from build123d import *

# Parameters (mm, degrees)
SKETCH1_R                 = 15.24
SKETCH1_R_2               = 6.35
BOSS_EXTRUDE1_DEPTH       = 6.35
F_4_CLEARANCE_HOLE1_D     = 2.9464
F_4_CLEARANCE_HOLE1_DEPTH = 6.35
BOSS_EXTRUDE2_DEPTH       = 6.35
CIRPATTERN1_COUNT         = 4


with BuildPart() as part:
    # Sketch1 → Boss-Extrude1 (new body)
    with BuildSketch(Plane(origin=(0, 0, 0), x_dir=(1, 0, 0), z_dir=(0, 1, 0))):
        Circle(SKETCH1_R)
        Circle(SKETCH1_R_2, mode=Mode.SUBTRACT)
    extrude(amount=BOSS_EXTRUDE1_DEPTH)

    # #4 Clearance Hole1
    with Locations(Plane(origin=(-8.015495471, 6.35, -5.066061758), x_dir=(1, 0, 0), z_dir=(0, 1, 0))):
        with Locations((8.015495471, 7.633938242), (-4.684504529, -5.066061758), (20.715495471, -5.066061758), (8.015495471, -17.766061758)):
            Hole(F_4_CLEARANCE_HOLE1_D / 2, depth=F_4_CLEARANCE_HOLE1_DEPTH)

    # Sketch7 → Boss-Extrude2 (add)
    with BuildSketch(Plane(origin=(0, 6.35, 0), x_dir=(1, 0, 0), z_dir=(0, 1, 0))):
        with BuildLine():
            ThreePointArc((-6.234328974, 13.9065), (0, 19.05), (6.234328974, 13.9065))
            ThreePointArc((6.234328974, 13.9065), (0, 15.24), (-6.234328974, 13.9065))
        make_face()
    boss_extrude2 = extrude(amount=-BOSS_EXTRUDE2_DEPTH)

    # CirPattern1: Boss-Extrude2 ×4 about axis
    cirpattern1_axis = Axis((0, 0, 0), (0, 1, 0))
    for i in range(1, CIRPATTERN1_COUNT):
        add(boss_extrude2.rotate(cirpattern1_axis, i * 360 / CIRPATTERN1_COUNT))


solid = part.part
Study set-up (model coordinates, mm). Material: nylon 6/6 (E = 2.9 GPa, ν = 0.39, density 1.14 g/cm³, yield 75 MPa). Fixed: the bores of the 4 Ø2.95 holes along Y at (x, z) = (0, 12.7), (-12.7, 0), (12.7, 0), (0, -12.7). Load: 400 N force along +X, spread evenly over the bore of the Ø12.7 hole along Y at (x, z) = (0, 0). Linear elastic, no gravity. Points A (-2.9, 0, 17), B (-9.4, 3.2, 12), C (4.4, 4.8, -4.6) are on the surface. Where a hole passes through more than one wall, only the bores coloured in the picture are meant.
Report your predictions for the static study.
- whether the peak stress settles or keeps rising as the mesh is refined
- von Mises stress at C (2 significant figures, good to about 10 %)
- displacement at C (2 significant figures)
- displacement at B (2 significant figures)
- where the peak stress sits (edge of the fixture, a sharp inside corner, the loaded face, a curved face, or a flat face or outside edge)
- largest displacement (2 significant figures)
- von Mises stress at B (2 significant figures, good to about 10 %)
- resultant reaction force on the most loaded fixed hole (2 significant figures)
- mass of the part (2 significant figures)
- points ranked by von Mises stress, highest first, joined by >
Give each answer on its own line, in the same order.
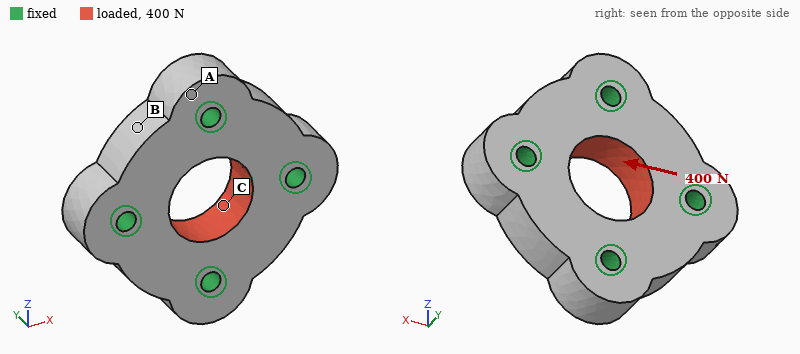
keeps rising
2.2 MPa
7.2 µm
4.0 µm
edge of the fixture
7.8 µm
1.1 MPa
120 N
5.2 g
C > B > A
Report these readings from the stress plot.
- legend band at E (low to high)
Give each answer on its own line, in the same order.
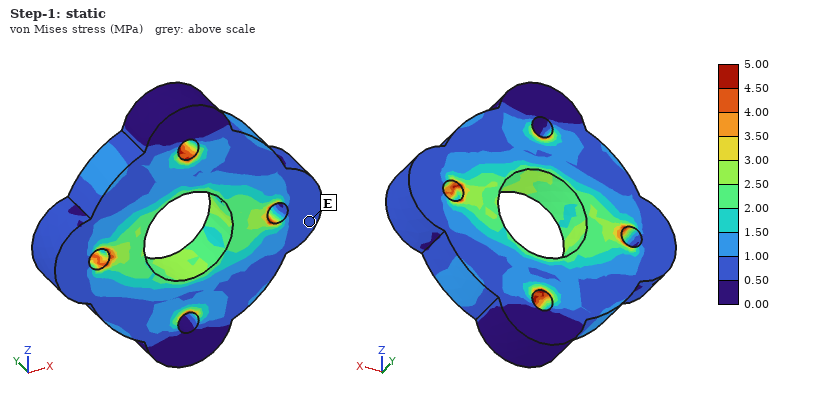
0.50 to 1.00 MPa
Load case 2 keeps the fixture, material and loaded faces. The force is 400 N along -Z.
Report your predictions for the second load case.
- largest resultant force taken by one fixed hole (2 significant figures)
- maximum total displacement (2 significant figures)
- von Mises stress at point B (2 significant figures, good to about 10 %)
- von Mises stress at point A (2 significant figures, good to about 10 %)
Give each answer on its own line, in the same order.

120 N
7.9 µm
1.0 MPa
0.63 MPa
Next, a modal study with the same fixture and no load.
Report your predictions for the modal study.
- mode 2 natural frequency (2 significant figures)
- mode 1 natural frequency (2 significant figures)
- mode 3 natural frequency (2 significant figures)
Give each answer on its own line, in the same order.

19 kHz
18 kHz
19 kHz
